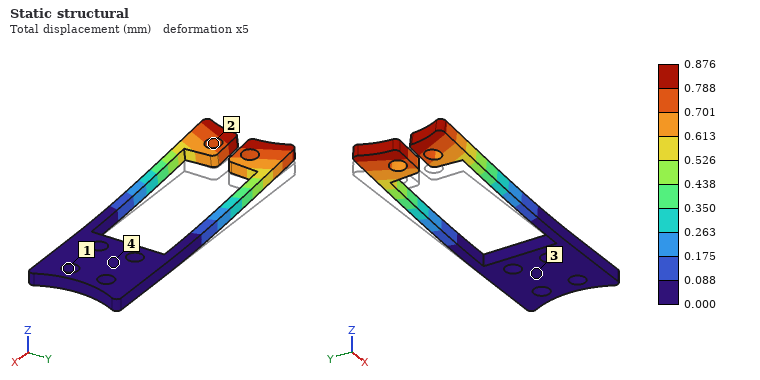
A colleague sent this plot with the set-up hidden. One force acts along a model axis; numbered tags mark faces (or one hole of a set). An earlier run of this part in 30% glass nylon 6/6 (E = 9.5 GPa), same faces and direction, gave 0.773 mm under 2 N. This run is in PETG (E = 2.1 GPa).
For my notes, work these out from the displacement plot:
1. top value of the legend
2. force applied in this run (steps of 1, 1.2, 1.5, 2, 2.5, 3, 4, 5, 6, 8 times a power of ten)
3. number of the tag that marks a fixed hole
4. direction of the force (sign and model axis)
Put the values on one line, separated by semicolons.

0.876 mm; 0.5 N; 1; +Z
